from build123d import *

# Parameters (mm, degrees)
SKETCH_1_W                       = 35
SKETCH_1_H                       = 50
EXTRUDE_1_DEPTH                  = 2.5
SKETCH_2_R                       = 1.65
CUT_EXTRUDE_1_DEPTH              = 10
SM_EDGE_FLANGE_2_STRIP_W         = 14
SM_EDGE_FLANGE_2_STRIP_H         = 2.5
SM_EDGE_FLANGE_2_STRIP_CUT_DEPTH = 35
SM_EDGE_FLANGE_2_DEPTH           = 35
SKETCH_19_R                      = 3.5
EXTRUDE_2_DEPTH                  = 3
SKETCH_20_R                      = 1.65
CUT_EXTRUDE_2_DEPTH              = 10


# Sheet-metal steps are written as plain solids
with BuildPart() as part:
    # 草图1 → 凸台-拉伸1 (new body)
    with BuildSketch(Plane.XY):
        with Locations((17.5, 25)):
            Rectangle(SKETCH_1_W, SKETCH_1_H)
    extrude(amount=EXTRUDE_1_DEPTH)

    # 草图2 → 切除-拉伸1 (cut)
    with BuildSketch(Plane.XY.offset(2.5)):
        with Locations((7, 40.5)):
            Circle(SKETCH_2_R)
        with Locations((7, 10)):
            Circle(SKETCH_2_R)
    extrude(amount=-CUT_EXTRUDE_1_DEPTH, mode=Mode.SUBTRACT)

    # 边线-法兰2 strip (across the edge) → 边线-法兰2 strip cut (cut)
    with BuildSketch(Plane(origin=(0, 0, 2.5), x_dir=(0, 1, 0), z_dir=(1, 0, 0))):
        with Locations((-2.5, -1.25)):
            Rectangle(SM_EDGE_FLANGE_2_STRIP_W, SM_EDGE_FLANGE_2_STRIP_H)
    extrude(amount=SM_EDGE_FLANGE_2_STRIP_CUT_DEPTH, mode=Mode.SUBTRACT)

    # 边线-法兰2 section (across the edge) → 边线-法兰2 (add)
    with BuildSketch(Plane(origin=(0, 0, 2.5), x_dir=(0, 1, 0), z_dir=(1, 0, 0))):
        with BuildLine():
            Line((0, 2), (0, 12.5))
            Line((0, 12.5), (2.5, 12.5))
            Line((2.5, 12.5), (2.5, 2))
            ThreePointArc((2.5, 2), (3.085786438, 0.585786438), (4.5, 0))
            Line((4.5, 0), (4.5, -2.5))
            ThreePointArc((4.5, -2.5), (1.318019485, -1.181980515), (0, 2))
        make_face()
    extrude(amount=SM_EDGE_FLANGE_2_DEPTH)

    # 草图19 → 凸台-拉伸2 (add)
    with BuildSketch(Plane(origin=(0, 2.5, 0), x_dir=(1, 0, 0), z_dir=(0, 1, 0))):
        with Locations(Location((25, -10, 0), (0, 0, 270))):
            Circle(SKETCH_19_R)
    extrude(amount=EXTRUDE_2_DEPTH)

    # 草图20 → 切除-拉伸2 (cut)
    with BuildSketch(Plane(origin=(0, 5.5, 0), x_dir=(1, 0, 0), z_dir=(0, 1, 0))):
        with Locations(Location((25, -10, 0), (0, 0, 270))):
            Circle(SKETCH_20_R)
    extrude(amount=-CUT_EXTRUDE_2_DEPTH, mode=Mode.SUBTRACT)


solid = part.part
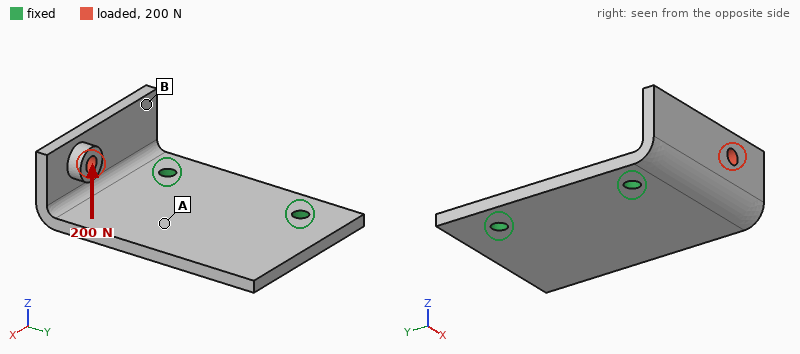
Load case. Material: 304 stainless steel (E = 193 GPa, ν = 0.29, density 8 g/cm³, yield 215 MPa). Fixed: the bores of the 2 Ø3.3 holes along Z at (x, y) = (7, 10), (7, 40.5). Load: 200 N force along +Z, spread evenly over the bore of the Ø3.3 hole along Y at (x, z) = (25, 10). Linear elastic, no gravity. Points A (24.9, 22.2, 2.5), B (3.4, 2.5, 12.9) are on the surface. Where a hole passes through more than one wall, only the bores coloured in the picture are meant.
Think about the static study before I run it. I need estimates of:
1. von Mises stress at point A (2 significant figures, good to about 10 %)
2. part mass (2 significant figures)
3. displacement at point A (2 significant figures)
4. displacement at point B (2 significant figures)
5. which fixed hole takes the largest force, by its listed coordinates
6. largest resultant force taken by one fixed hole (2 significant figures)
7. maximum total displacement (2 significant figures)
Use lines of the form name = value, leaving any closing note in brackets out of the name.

von Mises stress at point A = 26 MPa
part mass = 43 g
displacement at point A = 21 µm
displacement at point B = 34 µm
which fixed hole takes the largest force, by its listed coordinates = (7, 10)
largest resultant force taken by one fixed hole = 220 N
maximum total displacement = 95 µm
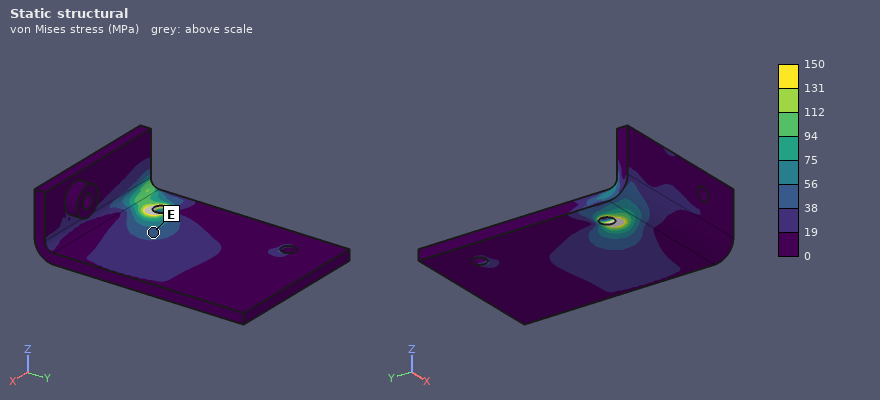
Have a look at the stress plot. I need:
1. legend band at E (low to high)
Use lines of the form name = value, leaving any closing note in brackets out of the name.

legend band at E = 38 to 56 MPa
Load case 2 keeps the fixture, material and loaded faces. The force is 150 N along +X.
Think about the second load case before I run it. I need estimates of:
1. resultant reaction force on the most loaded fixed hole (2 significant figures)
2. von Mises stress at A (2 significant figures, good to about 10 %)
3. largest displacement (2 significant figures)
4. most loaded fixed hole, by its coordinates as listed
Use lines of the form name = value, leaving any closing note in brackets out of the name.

resultant reaction force on the most loaded fixed hole = 180 N
von Mises stress at A = 8.3 MPa
largest displacement = 35 µm
most loaded fixed hole, by its coordinates as listed = (7, 10)
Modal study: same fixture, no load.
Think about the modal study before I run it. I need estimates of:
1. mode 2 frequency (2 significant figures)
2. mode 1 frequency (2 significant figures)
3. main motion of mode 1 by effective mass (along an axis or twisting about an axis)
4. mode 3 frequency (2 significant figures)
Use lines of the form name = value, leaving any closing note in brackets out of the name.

mode 2 frequency = 3200 Hz
mode 1 frequency = 2400 Hz
main motion of mode 1 by effective mass = along Z
mode 3 frequency = 5000 Hz
